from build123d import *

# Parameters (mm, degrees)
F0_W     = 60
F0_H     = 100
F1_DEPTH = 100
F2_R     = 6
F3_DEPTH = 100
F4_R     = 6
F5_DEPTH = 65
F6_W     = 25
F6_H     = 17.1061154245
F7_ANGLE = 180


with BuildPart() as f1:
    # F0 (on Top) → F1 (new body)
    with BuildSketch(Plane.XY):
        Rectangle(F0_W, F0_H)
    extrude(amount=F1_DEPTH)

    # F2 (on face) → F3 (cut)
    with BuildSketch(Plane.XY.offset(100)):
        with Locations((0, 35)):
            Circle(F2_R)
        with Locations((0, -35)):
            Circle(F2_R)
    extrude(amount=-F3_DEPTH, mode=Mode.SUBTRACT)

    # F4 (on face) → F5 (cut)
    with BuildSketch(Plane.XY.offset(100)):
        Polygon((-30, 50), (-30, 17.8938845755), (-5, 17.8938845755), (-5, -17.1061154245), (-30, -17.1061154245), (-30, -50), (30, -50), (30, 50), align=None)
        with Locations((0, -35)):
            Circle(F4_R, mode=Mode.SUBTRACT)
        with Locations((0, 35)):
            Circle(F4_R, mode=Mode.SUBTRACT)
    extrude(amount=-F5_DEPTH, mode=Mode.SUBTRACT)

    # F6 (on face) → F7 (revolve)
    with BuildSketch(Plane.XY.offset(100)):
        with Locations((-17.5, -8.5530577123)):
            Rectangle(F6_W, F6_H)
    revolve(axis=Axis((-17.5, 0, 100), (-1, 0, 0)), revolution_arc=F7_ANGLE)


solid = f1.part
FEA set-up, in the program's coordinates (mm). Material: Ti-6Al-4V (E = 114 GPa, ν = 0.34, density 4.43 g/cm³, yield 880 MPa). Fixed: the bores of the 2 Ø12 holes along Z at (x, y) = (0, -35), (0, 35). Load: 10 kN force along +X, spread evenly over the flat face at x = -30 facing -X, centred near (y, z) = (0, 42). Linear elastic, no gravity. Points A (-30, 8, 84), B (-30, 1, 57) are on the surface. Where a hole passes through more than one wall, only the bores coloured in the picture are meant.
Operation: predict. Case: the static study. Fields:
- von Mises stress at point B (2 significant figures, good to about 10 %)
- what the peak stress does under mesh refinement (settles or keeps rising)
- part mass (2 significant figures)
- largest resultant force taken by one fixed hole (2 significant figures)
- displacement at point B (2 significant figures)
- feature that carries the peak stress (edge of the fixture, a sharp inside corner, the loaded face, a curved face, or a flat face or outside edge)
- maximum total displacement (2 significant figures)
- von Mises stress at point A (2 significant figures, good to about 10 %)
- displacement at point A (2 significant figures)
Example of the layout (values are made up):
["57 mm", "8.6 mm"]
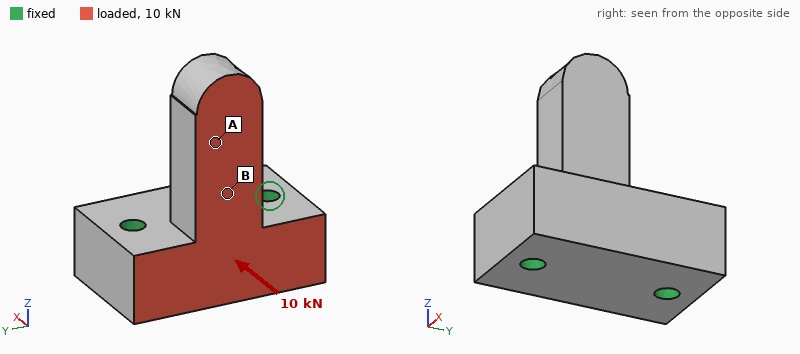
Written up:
["25 MPa", "keeps rising", "1.2 kg", "5.1 kN", "0.031 mm", "a sharp inside corner", "0.11 mm", "7.5 MPa", "0.063 mm"]
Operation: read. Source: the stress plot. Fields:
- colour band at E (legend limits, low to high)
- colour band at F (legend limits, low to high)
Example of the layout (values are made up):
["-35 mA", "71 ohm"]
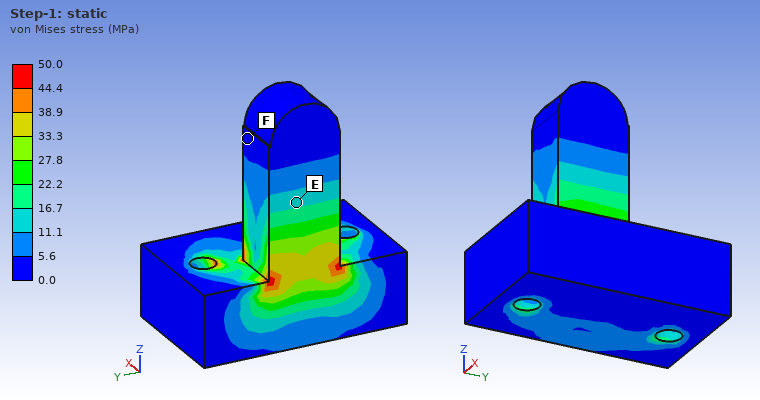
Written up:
["11.1 to 16.7 MPa", "0.0 to 5.6 MPa"]
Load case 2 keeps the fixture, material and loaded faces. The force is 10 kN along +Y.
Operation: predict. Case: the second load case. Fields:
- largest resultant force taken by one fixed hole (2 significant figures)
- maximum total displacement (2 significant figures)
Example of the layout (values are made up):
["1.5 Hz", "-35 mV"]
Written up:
["7.2 kN", "57 µm"]
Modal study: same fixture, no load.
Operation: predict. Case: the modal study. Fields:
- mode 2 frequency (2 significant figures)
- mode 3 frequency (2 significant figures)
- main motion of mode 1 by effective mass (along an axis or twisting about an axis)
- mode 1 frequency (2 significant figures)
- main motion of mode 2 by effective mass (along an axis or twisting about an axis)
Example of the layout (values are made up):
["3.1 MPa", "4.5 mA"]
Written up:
["3300 Hz", "8400 Hz", "along X", "2300 Hz", "along Y"]
